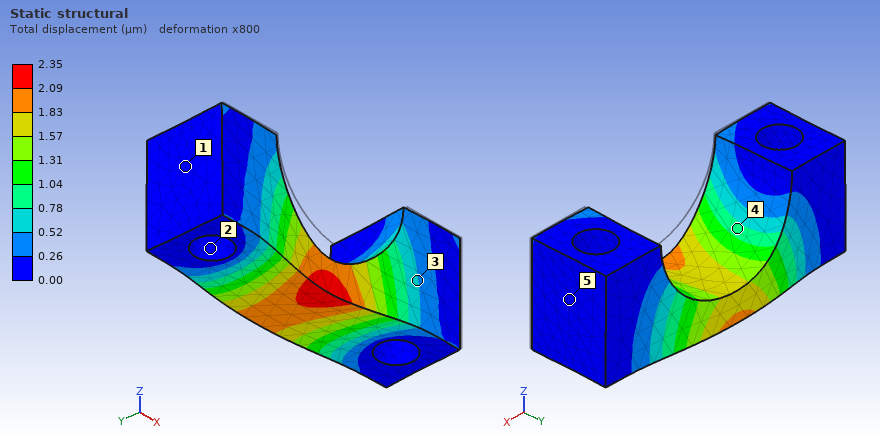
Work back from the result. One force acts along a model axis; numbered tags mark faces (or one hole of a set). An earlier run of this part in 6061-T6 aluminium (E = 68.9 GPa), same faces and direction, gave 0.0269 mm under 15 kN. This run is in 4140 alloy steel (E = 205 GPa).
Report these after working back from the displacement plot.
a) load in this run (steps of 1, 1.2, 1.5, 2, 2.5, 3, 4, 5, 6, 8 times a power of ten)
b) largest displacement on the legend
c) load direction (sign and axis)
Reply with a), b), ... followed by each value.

a) 4 kN
b) 2.35 µm
c) +Y
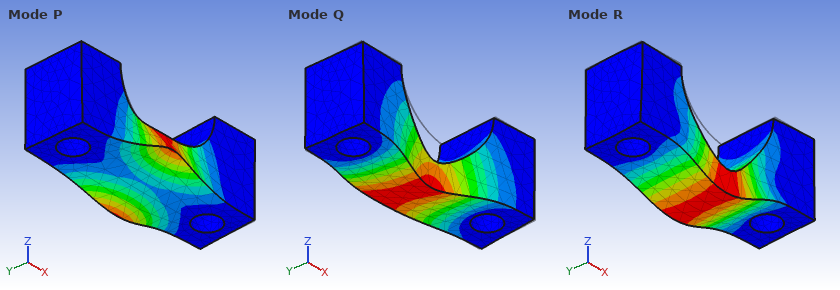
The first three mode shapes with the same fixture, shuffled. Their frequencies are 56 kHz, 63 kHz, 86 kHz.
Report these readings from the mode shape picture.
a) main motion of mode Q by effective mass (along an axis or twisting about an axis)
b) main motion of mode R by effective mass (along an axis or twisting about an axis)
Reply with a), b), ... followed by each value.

a) along Y
b) along Z
